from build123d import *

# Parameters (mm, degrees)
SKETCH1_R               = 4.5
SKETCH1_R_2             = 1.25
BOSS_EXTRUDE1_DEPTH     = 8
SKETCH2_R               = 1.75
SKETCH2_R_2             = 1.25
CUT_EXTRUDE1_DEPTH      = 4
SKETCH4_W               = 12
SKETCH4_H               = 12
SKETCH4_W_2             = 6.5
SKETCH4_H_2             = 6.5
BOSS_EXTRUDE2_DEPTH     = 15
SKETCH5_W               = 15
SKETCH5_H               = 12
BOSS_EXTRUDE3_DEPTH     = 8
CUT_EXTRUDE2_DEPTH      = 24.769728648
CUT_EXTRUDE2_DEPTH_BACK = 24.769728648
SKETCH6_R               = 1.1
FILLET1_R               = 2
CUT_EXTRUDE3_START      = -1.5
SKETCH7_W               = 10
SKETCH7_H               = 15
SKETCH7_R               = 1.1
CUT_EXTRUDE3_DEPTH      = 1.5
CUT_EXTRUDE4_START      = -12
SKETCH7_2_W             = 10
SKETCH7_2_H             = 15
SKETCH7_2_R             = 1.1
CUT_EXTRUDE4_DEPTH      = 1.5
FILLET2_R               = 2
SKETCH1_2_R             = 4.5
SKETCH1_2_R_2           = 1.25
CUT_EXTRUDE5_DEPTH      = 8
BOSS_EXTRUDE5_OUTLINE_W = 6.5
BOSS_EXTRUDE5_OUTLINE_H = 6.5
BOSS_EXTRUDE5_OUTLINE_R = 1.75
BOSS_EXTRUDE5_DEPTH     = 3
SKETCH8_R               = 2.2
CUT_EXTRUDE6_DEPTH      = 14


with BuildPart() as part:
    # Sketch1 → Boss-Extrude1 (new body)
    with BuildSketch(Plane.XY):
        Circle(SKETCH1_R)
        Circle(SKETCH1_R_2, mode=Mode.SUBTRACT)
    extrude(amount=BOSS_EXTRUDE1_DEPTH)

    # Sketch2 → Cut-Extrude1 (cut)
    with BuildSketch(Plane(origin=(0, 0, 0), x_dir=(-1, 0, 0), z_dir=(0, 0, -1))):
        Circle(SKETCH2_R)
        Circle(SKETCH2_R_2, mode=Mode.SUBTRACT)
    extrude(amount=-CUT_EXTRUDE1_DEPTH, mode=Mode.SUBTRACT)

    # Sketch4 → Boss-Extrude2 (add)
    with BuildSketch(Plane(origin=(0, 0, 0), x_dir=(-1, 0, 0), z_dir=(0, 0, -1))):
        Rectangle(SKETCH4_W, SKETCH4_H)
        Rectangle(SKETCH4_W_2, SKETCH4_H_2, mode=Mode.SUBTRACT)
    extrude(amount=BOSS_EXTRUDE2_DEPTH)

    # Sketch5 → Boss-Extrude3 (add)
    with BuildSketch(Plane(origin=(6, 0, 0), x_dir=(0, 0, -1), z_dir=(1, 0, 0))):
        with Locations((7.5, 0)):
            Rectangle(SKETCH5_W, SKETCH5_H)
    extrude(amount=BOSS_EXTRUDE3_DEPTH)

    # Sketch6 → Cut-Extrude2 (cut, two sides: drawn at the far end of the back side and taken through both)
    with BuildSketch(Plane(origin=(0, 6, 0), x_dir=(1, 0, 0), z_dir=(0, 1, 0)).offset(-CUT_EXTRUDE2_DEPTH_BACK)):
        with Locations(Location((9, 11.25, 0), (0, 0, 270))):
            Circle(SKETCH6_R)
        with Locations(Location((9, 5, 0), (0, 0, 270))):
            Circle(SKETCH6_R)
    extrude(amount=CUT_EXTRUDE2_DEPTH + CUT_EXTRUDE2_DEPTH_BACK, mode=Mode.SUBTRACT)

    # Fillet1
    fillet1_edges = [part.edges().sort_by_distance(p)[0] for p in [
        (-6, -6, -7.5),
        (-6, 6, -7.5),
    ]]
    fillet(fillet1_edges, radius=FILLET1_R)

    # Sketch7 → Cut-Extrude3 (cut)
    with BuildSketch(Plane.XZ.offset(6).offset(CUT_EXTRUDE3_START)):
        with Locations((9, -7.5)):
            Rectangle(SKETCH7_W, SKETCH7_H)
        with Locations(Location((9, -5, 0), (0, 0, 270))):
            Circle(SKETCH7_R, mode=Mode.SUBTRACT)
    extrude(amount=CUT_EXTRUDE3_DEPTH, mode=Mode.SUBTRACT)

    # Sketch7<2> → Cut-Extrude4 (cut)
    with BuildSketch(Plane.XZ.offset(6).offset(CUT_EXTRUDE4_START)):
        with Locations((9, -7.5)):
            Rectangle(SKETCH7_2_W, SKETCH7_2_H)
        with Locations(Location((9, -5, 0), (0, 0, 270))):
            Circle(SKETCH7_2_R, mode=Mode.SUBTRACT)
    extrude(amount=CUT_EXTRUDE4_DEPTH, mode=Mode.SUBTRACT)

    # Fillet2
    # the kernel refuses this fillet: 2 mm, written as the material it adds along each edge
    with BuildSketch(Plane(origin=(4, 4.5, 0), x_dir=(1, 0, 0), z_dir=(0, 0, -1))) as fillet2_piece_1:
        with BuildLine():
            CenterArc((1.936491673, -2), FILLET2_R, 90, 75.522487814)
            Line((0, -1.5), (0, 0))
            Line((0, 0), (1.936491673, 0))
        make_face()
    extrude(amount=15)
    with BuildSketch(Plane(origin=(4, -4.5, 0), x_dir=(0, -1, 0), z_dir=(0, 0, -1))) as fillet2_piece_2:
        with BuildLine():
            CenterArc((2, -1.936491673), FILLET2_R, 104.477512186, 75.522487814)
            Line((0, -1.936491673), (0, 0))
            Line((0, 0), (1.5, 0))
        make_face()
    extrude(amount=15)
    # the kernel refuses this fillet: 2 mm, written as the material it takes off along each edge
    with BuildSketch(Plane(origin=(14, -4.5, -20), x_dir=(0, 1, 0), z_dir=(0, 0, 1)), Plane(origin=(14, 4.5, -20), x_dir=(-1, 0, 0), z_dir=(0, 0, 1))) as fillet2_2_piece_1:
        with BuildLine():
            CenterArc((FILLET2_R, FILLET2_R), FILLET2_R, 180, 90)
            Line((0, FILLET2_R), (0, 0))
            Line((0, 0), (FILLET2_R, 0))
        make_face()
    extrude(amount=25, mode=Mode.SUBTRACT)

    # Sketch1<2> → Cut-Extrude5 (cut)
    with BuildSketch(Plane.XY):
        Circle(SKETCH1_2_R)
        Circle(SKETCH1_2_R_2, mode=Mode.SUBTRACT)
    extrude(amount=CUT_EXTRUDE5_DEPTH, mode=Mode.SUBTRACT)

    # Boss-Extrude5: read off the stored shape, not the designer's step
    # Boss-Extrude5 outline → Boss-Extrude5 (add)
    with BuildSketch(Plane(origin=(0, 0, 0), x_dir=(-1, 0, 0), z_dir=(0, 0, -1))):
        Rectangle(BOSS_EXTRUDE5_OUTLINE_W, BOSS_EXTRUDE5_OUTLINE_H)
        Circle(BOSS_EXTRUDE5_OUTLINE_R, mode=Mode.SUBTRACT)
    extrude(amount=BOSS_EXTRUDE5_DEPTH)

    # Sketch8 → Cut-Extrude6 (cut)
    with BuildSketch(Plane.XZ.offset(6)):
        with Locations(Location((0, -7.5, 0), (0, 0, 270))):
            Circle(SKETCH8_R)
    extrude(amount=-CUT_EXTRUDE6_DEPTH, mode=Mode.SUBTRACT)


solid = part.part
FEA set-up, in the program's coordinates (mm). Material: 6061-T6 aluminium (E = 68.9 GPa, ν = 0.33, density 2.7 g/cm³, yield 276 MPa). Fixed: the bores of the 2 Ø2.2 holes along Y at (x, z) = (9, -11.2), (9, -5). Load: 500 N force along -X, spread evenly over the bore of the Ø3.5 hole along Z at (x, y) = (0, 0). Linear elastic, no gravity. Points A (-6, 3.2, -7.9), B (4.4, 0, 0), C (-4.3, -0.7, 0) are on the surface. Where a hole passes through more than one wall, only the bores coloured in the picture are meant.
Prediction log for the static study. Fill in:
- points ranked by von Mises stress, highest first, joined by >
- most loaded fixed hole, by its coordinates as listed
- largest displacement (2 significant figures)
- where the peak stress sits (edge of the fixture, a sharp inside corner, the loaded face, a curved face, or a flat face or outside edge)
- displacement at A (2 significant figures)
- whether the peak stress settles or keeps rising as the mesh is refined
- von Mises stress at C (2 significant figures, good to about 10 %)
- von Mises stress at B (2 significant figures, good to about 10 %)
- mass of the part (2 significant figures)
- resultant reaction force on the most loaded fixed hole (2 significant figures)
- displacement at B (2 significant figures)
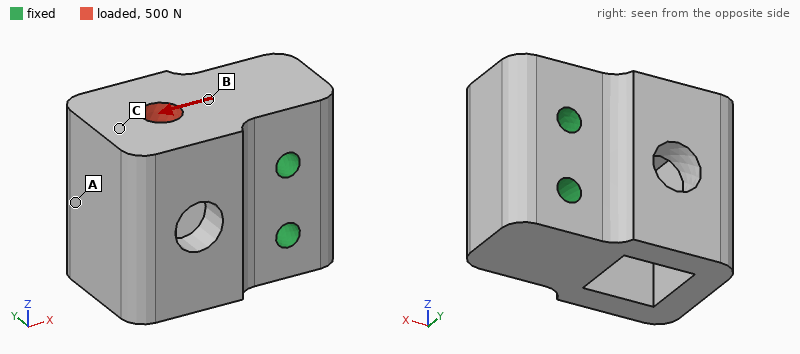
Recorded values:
B > C > A
(9, -5)
4.7 µm
edge of the fixture
3.1 µm
keeps rising
7.9 MPa
16 MPa
6.6 g
670 N
2.1 µm
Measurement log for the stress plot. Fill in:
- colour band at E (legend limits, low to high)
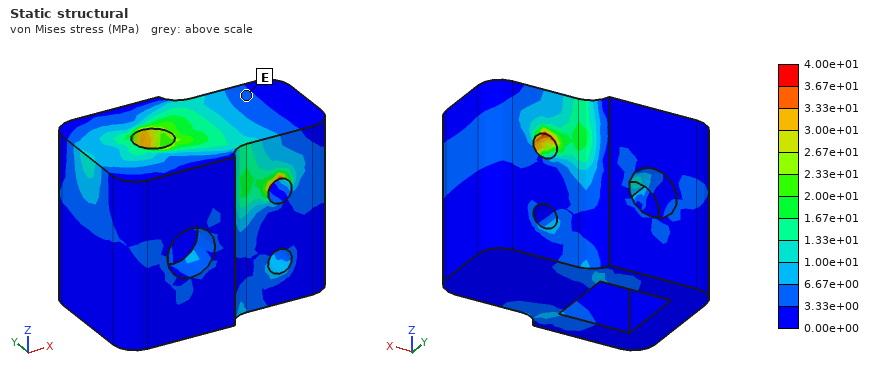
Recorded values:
3.33e+00 to 6.67e+00 MPa
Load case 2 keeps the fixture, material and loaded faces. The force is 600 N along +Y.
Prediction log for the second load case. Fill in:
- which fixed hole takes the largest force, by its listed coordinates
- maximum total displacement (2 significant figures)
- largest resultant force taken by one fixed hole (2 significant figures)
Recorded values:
(9, -5)
15 µm
570 N
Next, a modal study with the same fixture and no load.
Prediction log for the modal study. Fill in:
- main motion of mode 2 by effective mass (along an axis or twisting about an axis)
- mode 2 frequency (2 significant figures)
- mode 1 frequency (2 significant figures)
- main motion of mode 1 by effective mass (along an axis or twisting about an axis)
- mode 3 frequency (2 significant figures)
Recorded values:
along Z
24 kHz
18 kHz
along Y
35 kHz
